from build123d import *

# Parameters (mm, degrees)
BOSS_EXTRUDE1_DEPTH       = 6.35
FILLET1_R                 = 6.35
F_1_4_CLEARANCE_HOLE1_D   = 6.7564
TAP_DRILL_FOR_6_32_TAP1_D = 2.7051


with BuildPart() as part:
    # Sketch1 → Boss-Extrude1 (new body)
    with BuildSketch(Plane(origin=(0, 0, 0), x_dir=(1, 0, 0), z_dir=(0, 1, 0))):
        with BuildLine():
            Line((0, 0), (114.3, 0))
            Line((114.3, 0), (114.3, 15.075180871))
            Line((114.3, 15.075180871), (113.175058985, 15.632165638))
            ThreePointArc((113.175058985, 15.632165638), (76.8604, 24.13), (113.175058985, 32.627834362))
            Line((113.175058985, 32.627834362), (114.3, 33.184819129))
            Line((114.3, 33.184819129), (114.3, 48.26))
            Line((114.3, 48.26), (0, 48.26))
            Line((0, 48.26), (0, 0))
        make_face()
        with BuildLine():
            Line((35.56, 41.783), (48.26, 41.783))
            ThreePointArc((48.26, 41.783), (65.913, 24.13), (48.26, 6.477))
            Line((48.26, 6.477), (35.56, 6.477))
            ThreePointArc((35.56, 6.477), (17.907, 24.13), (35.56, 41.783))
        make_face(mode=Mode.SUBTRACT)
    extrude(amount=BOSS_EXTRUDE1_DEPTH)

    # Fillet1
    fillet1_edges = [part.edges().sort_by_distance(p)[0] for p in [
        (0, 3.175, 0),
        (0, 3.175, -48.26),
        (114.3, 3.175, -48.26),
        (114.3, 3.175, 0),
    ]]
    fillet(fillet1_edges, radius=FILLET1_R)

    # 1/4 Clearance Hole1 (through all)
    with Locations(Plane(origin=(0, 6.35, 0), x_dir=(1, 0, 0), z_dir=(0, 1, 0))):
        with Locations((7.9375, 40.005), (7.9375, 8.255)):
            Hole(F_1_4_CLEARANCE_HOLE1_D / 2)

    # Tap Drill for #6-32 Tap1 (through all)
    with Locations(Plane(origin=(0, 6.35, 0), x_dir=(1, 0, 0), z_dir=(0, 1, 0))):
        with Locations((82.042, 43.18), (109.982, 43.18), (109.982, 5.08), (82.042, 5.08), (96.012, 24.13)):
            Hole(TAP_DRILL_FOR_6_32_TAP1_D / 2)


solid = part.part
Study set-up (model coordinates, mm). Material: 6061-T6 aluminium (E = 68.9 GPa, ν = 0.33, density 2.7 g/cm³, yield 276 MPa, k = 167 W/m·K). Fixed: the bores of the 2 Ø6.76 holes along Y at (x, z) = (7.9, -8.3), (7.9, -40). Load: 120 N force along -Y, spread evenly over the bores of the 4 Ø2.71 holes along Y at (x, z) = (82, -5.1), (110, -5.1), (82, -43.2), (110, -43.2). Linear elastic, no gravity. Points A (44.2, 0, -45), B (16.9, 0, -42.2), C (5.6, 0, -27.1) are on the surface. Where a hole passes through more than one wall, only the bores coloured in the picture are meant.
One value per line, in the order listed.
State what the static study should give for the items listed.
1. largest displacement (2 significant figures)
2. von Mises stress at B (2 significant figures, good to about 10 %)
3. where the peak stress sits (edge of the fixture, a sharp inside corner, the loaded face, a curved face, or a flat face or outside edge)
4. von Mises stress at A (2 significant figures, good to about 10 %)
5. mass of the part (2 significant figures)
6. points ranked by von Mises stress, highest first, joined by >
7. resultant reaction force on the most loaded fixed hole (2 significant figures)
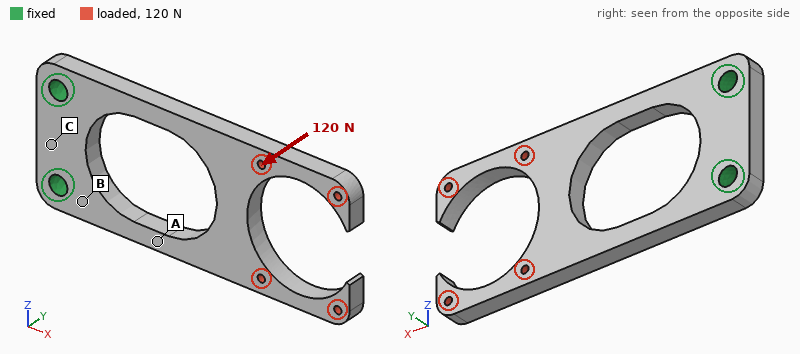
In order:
1.3 mm
48 MPa
a curved face
73 MPa
48 g
A > B > C
60 N
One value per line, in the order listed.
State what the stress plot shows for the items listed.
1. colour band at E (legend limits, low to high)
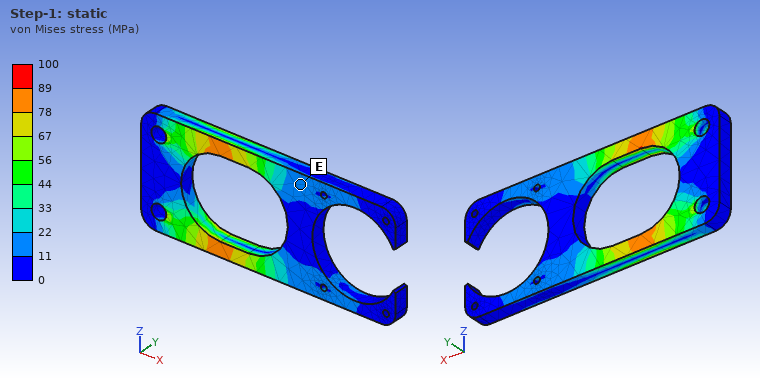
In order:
11 to 22 MPa
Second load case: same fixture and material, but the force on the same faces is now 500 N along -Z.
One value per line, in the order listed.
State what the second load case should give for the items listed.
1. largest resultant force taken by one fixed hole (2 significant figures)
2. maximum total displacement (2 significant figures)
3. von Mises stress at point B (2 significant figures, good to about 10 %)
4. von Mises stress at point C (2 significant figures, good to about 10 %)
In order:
1.1 kN
0.33 mm
15 MPa
5.7 MPa
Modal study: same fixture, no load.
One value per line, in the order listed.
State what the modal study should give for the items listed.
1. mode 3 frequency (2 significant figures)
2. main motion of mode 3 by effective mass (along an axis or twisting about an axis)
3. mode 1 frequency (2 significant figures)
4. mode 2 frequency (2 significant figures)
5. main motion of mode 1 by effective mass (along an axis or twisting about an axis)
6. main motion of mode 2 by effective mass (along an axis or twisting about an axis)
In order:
1900 Hz
along Z
470 Hz
1300 Hz
along Y
twisting about X
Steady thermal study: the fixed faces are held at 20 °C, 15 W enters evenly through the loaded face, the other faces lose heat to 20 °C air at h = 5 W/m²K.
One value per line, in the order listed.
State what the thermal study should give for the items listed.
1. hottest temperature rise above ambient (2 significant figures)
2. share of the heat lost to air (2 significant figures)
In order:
67 K
9.2 %
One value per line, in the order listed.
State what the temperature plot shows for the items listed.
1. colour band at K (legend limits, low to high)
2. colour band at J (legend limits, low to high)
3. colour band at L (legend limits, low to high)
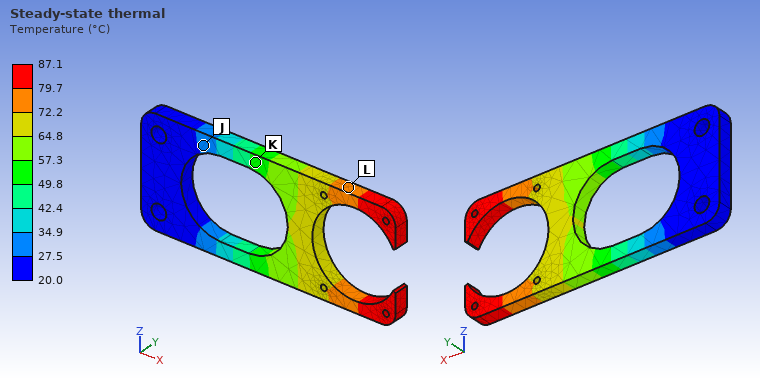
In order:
49.8 to 57.3 °C
27.5 to 34.9 °C
72.2 to 79.7 °C
